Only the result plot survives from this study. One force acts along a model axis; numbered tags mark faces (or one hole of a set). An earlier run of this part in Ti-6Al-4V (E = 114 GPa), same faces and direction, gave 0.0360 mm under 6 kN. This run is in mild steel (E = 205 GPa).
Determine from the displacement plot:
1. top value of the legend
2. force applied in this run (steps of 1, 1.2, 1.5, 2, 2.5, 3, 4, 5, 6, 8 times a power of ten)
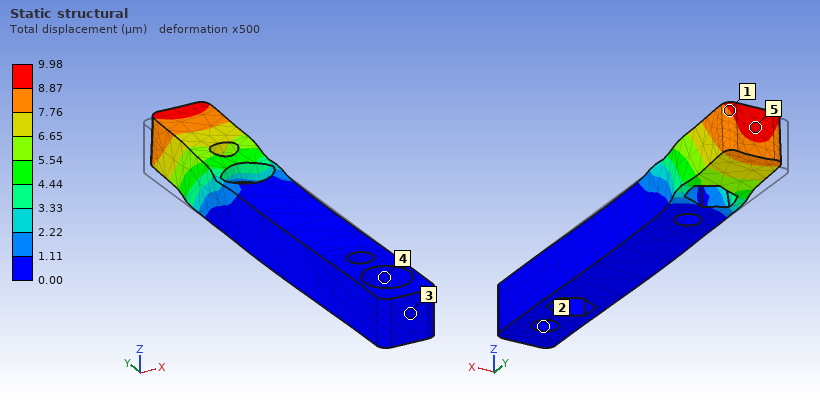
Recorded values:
9.98 µm
3 kN
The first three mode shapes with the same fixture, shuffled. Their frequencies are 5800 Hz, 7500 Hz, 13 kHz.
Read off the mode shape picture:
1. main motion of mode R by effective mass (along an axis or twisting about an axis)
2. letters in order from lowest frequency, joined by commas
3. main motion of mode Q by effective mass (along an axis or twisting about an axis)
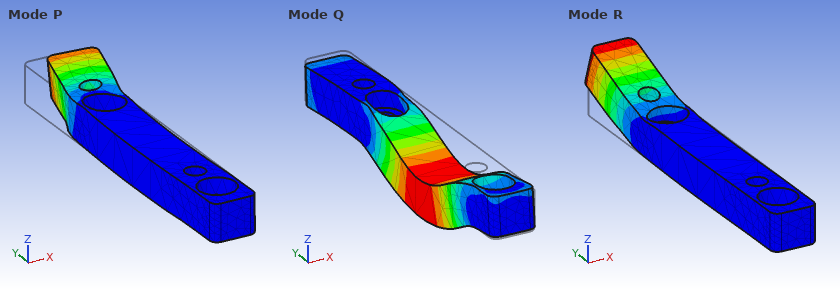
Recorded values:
along Z
R, P, Q
along Z
